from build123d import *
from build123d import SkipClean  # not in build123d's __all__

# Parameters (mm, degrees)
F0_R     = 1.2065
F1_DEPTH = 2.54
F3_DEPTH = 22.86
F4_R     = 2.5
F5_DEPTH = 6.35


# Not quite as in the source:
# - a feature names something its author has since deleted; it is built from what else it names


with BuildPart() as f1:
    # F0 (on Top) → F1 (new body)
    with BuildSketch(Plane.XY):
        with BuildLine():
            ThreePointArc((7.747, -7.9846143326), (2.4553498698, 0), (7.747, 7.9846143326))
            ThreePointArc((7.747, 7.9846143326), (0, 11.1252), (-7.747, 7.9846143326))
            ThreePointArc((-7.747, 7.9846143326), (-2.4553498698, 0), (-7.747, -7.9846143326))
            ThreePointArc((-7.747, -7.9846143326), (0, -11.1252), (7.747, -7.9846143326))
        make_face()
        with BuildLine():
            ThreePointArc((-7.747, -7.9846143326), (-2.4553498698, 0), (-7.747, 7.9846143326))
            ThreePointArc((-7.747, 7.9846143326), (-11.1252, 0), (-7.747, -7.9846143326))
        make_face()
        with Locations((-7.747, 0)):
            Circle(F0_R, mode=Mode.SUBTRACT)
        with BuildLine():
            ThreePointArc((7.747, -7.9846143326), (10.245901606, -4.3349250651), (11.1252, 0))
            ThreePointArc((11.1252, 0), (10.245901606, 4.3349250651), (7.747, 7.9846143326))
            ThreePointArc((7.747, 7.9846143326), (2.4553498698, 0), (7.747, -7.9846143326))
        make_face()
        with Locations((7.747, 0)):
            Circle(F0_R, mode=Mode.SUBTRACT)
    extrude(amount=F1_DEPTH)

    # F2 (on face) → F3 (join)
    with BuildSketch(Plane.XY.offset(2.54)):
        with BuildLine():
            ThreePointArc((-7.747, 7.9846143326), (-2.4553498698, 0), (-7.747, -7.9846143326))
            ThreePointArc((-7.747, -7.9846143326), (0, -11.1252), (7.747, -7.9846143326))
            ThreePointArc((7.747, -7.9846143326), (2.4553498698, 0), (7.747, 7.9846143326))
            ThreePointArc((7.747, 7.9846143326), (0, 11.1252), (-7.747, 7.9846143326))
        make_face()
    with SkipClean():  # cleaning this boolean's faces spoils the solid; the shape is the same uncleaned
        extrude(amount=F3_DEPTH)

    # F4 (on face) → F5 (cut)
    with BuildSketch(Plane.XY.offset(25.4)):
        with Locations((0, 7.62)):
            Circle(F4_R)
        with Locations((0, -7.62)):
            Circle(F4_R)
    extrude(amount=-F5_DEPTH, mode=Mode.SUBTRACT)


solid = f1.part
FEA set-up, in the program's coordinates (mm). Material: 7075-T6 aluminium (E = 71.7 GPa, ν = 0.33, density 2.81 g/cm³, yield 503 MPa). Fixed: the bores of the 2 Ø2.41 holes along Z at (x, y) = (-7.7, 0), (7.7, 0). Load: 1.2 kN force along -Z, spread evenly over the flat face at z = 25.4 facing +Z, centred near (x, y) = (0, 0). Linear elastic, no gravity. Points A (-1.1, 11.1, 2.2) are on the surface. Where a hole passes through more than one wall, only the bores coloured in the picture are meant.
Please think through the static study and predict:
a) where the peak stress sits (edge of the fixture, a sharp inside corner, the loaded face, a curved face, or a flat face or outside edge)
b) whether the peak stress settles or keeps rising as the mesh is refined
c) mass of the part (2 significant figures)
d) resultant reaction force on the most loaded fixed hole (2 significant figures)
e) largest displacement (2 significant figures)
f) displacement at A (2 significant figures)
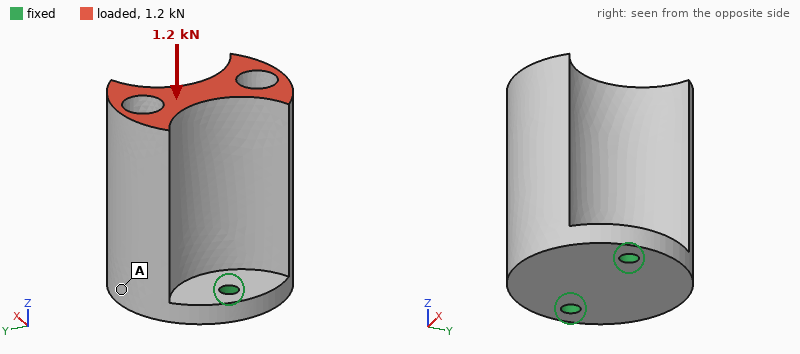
edge of the fixture
keeps rising
14 g
620 N
15 µm
13 µm
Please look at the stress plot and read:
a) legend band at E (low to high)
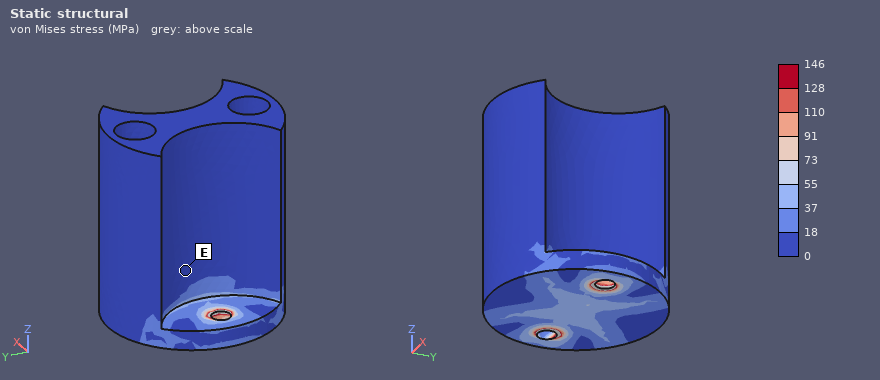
0 to 18 MPa
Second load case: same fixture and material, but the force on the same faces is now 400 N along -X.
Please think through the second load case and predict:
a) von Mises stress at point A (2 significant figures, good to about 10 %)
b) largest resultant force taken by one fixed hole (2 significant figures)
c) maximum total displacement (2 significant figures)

21 MPa
750 N
82 µm
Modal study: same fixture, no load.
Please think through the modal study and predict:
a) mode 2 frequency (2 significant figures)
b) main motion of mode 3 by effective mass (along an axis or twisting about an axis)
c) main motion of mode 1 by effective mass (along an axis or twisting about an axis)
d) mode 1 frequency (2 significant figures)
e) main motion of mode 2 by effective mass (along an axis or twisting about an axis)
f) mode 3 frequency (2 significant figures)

5900 Hz
along Z
along Y
3200 Hz
along X
13 kHz
